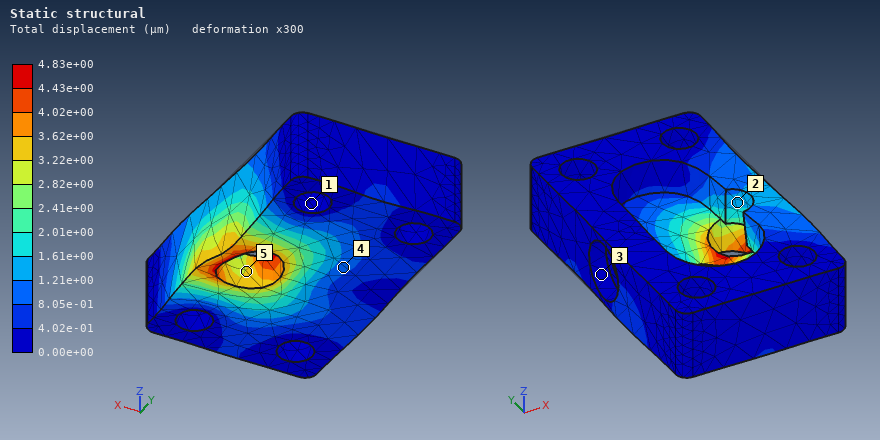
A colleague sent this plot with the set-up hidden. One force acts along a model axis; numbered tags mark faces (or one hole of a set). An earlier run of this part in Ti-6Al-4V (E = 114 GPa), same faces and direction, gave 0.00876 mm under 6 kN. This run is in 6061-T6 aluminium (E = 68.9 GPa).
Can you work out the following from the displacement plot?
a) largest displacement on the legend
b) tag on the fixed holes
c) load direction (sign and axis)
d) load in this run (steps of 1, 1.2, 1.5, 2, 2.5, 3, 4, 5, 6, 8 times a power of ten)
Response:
4.83e+00 µm
1
-Y
2 kN
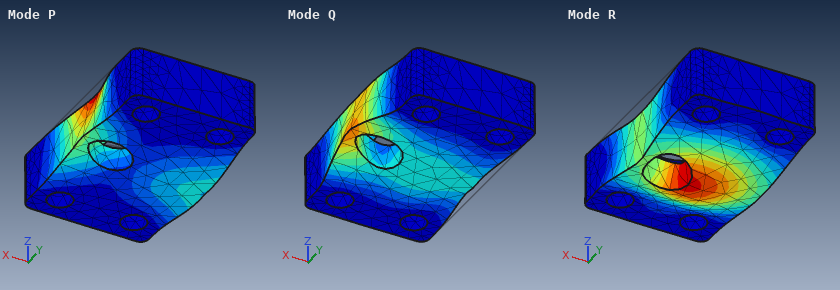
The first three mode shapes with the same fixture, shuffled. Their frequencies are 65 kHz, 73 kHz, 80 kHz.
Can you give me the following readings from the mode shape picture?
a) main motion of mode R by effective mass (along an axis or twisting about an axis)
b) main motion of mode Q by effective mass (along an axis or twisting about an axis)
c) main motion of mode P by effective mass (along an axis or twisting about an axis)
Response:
along Z
along X
along X
